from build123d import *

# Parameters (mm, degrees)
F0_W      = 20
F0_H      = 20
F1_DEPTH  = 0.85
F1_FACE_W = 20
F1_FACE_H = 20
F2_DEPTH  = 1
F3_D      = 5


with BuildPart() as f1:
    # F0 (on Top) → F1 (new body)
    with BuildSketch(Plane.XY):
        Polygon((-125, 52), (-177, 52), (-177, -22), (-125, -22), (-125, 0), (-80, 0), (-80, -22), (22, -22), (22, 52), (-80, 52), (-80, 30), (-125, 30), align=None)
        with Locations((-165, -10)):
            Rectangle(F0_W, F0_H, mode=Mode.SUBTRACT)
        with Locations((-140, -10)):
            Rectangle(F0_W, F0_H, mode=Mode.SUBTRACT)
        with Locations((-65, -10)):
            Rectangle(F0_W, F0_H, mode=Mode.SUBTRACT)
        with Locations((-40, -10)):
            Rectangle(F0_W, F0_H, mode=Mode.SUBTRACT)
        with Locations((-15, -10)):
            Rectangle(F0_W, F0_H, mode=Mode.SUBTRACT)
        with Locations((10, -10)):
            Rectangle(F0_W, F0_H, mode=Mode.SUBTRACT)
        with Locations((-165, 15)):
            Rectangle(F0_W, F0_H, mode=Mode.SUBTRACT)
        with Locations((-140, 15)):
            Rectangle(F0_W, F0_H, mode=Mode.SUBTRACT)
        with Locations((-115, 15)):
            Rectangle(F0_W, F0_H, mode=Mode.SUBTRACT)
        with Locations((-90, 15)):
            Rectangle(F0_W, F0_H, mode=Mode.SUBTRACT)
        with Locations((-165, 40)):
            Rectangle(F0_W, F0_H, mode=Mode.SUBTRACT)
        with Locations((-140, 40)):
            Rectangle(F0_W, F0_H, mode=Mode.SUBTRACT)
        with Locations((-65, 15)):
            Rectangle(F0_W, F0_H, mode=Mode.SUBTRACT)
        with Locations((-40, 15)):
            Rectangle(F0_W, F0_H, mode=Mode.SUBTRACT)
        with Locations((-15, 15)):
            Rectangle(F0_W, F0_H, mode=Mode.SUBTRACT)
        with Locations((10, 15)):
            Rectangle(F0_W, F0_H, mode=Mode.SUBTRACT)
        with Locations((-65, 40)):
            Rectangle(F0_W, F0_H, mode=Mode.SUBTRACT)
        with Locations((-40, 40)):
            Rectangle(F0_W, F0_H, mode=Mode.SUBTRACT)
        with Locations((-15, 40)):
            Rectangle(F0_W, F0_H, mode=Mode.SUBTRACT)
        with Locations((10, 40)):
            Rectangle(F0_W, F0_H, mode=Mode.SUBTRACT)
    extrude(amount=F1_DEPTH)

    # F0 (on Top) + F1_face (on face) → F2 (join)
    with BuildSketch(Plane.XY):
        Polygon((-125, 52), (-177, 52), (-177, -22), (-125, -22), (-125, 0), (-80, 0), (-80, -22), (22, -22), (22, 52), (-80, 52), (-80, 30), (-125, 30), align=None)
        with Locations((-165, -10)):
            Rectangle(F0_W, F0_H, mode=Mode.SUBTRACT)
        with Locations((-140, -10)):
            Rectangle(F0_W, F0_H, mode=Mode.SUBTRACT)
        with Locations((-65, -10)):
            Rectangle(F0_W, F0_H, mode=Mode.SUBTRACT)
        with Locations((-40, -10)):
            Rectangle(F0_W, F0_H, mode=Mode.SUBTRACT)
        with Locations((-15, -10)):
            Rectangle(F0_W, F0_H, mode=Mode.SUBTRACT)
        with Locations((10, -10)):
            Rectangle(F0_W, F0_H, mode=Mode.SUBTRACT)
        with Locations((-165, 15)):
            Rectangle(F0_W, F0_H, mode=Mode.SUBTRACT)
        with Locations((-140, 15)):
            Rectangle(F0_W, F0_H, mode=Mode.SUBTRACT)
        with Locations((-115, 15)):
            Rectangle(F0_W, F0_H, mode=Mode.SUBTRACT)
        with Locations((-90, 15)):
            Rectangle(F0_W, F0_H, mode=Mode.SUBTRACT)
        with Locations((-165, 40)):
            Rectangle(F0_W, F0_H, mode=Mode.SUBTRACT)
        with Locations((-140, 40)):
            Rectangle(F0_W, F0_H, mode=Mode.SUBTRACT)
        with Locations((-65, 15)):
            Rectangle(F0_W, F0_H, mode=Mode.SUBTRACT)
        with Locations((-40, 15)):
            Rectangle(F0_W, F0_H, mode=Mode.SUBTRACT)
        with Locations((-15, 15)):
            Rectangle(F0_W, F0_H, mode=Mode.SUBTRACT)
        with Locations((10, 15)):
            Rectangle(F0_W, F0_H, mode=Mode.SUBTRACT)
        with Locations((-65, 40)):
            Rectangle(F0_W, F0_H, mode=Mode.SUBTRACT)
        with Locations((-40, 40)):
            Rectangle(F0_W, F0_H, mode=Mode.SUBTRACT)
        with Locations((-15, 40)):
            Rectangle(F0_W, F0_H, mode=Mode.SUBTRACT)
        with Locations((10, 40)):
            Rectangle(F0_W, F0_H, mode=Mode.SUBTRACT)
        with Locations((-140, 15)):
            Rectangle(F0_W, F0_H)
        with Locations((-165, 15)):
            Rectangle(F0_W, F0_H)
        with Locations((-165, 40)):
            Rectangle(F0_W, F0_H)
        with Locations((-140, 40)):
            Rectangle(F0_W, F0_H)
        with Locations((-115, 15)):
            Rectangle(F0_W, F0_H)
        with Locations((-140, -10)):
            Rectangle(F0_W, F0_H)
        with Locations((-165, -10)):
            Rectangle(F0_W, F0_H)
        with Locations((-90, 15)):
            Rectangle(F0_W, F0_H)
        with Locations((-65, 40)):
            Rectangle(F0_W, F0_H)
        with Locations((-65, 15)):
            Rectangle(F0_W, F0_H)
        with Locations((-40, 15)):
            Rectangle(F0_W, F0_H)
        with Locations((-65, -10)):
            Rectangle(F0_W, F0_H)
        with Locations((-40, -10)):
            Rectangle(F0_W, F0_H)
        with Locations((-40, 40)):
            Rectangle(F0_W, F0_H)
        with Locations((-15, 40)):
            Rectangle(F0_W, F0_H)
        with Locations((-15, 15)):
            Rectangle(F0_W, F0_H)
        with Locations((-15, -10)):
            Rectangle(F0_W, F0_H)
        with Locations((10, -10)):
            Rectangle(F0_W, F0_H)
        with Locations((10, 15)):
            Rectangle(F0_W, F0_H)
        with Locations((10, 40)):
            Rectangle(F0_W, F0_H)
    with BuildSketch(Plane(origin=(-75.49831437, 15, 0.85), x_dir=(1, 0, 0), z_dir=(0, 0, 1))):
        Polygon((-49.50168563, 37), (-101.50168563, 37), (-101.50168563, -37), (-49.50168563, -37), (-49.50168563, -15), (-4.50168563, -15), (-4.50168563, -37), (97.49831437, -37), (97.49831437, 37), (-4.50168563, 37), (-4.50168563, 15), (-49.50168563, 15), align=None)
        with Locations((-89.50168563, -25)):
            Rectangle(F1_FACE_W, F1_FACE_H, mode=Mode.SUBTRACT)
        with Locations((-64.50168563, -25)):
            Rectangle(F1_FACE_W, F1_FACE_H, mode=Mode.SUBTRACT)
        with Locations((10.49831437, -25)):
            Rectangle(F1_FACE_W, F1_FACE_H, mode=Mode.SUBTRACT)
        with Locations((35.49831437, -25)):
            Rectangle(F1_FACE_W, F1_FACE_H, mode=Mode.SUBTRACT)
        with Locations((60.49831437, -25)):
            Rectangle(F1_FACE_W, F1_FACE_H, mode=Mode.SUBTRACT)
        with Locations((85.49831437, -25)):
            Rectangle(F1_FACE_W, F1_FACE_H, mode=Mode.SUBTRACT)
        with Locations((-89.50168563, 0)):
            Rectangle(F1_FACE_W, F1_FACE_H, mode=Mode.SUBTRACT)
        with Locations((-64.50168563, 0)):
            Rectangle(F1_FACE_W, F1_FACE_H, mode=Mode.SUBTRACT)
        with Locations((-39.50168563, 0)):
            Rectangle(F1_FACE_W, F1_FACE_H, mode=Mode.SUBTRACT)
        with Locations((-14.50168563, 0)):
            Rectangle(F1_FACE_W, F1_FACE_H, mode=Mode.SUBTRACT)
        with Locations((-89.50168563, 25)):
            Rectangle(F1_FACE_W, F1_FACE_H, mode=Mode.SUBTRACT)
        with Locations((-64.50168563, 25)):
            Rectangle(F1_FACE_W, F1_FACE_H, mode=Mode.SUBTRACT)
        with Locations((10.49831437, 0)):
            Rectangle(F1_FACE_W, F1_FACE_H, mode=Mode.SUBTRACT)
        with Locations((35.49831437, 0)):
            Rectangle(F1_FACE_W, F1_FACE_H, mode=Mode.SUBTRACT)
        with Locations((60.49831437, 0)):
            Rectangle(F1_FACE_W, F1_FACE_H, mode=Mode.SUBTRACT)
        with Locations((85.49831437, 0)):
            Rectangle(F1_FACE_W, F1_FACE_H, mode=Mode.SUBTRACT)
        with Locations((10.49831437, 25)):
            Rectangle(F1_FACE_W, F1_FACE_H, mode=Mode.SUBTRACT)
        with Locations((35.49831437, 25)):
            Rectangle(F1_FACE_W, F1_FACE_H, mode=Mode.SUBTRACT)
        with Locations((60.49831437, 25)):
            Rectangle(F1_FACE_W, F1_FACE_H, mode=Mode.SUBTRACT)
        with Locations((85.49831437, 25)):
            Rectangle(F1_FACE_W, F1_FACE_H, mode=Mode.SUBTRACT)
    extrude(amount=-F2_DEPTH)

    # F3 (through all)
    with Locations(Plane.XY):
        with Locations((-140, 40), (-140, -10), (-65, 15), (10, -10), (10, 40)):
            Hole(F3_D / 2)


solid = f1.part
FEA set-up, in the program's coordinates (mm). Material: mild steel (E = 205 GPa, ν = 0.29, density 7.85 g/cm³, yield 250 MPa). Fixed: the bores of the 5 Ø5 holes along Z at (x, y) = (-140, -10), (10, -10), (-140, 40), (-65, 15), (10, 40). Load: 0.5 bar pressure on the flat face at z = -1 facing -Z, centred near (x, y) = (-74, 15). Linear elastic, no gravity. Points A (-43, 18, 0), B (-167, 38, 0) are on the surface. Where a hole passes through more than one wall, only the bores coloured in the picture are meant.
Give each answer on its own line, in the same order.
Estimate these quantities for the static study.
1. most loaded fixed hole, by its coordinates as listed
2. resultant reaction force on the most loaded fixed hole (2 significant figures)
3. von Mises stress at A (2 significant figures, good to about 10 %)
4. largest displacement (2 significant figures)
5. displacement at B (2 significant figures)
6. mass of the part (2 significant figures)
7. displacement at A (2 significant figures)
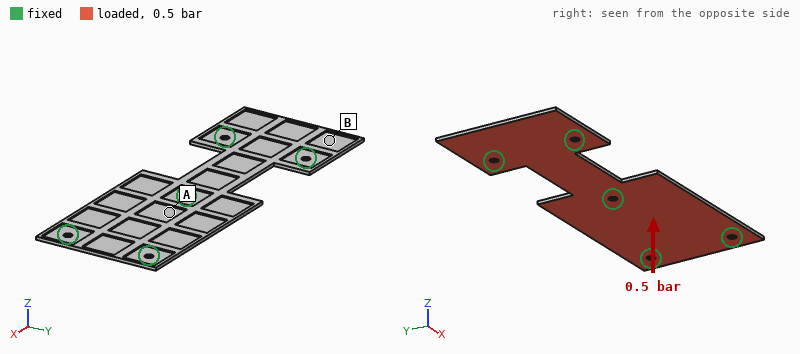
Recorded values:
(-65, 15)
280 N
35 MPa
0.35 mm
0.22 mm
130 g
0.11 mm
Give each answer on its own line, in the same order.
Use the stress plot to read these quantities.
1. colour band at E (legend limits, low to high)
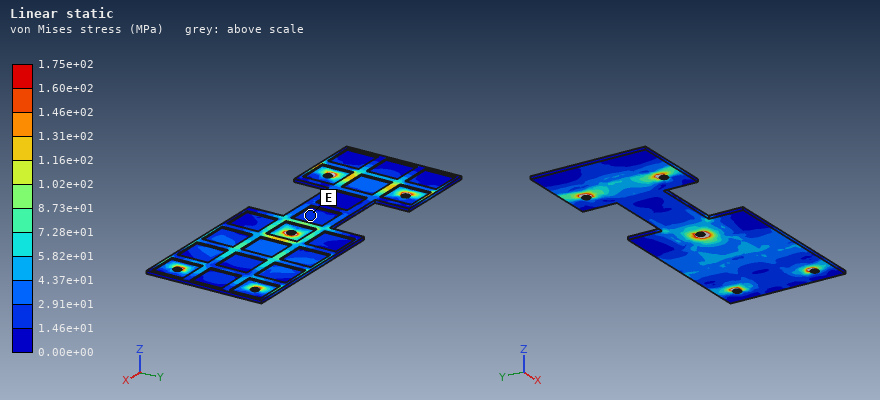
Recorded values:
1.46e+01 to 2.91e+01 MPa
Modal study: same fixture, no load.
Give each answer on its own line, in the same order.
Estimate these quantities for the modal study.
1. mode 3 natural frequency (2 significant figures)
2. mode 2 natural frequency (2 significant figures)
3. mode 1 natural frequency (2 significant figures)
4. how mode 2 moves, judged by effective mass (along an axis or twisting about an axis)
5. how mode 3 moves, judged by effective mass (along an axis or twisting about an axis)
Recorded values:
900 Hz
740 Hz
710 Hz
twisting about X
along Z
